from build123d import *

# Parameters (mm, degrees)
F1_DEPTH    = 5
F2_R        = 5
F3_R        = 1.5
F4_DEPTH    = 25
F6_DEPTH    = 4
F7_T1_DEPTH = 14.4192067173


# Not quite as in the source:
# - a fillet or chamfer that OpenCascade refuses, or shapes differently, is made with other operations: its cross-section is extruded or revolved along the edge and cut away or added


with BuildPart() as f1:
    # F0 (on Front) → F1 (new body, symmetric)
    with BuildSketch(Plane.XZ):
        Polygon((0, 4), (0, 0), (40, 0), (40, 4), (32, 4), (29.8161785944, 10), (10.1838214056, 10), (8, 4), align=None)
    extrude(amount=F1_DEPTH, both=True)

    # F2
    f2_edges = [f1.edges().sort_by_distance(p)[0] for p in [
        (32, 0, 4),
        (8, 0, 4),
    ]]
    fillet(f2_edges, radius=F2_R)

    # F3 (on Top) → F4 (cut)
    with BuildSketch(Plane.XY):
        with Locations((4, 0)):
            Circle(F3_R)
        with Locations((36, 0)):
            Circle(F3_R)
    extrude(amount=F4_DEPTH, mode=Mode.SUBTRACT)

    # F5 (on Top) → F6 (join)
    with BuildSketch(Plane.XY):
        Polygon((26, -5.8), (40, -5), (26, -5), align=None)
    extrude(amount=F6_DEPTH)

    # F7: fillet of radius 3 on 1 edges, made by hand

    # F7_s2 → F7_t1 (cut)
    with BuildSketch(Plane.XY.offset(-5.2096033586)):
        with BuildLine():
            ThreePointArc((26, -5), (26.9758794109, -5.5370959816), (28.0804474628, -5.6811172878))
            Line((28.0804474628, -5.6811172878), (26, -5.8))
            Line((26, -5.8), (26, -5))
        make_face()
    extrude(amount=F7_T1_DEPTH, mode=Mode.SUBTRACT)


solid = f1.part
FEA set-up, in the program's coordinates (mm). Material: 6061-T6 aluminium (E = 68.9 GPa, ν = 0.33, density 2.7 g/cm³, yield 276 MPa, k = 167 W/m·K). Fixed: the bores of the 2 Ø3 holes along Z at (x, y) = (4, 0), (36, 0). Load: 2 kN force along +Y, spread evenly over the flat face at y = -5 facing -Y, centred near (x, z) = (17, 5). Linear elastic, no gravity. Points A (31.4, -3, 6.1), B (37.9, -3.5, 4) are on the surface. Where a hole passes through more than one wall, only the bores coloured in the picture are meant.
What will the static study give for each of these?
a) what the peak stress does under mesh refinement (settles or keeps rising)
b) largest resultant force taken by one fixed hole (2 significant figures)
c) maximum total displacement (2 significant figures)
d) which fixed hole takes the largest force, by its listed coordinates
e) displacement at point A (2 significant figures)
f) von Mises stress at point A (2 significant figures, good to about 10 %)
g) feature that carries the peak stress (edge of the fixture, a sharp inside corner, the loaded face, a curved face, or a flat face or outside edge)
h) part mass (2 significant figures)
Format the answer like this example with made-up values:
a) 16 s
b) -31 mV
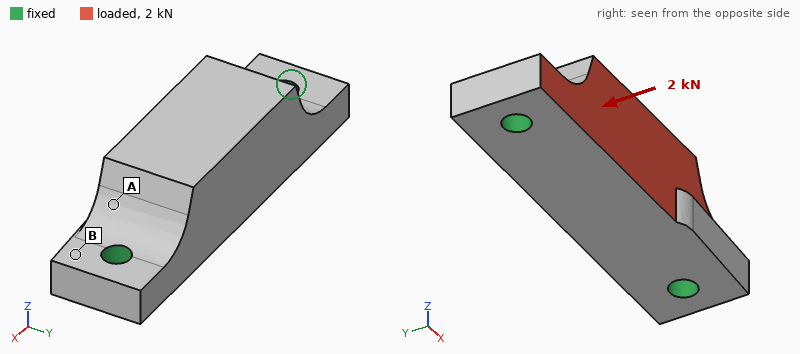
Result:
a) keeps rising
b) 1.2 kN
c) 35 µm
d) (4, 0)
e) 17 µm
f) 54 MPa
g) edge of the fixture
h) 7.9 g
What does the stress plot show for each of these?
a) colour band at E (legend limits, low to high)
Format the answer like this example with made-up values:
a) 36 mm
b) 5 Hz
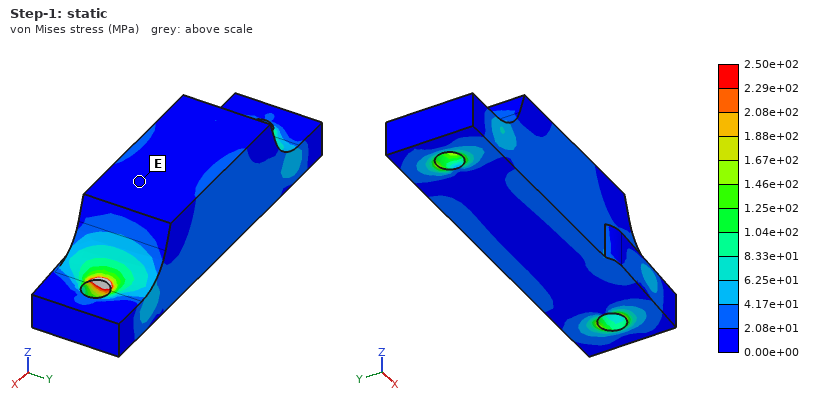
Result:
a) 0.00e+00 to 2.08e+01 MPa
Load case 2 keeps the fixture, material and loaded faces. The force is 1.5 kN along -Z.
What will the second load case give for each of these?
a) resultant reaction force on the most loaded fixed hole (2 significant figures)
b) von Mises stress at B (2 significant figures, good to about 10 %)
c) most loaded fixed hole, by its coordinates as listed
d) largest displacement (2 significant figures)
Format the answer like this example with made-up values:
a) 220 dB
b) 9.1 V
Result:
a) 1.0 kN
b) 26 MPa
c) (4, 0)
d) 37 µm
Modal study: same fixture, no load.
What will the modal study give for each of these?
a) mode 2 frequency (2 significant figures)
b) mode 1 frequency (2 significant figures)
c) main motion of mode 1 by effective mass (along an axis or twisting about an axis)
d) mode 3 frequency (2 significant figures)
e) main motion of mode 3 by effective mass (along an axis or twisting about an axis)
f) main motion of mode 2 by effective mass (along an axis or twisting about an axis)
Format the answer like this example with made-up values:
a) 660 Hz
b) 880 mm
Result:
a) 24 kHz
b) 17 kHz
c) along Y
d) 30 kHz
e) along Y
f) along Z
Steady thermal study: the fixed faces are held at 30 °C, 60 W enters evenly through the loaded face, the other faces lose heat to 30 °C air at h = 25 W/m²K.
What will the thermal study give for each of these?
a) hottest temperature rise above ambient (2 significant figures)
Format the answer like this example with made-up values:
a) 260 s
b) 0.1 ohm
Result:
a) 34 K
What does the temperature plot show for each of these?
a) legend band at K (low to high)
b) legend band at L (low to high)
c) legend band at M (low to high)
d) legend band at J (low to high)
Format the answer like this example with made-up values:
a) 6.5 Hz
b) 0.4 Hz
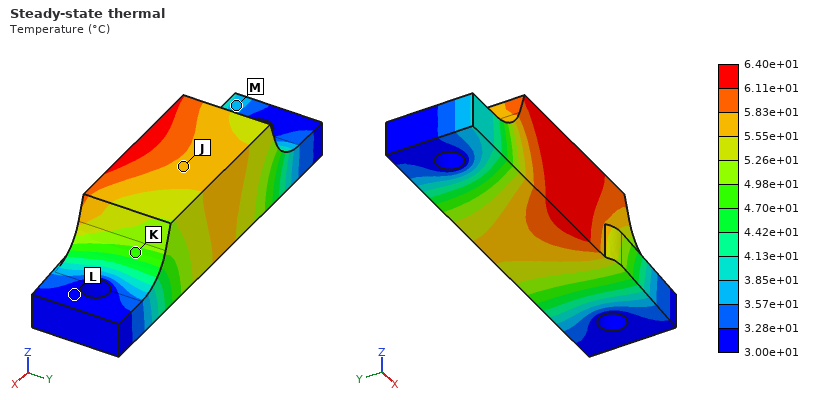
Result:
a) 4.70e+01 to 4.98e+01 °C
b) 3.00e+01 to 3.28e+01 °C
c) 3.57e+01 to 3.85e+01 °C
d) 5.55e+01 to 5.83e+01 °C
